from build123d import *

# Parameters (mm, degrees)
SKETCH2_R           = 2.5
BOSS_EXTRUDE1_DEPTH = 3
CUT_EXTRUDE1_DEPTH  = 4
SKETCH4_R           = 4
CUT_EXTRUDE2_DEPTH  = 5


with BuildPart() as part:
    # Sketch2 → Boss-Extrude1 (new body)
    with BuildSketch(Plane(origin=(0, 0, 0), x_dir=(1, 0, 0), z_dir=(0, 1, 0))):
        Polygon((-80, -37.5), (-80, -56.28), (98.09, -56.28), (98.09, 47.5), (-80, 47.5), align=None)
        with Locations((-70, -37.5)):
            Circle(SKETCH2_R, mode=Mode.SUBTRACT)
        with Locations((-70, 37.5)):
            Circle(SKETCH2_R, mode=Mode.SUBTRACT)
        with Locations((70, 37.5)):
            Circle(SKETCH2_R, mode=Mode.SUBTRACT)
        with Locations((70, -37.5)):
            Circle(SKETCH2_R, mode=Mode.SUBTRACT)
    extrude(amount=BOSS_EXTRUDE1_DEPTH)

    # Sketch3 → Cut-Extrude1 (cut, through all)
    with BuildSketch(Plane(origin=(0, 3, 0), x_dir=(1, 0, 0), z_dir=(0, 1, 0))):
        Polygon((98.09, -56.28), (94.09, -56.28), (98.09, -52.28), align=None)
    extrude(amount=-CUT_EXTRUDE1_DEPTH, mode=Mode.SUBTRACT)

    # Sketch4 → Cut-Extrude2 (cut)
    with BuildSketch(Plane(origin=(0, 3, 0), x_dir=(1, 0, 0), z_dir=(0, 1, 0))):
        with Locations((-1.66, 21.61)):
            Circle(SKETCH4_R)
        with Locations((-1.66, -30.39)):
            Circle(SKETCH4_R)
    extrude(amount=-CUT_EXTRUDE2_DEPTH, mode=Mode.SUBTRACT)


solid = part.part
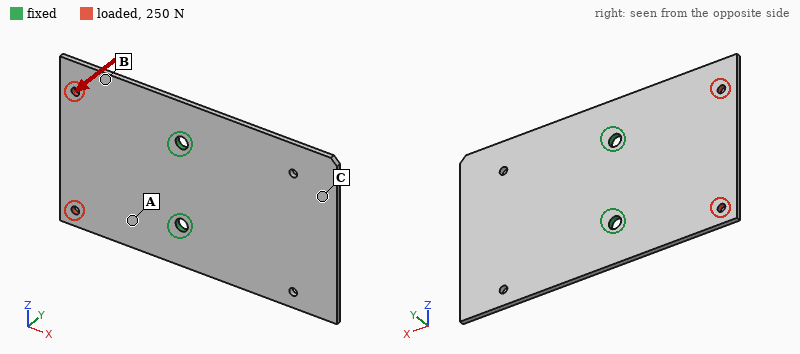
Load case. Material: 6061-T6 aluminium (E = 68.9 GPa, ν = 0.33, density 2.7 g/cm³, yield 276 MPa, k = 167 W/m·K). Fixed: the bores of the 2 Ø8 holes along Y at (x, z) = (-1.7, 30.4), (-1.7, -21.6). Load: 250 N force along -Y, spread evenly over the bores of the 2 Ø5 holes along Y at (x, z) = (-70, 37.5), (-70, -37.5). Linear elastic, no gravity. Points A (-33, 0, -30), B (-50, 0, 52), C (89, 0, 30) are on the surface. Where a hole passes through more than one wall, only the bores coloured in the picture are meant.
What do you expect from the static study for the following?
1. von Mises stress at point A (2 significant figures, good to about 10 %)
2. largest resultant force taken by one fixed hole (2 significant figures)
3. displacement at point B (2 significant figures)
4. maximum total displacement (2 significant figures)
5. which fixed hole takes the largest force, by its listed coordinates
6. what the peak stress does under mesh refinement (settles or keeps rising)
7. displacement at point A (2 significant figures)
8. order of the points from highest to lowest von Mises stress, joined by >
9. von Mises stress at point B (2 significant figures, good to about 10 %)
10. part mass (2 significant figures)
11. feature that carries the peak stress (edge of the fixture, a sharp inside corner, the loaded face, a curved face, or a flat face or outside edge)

55 MPa
140 N
0.85 mm
2.0 mm
(-1.7, -21.6)
keeps rising
0.44 mm
A > B > C
32 MPa
150 g
edge of the fixture
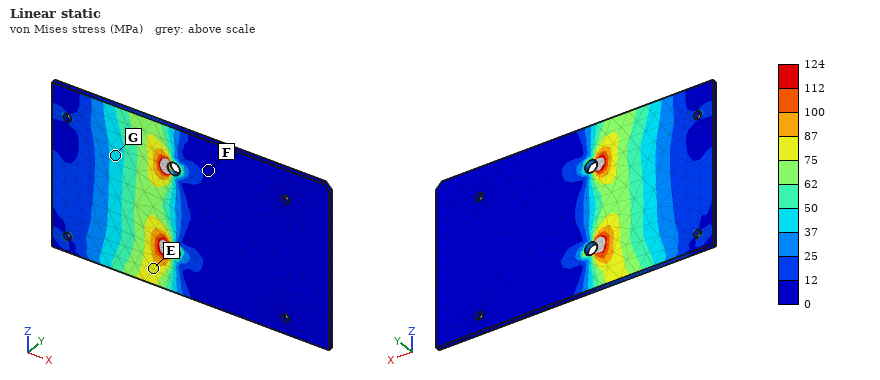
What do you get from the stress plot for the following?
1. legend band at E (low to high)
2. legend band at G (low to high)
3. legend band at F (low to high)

75 to 87 MPa
37 to 50 MPa
0 to 12 MPa
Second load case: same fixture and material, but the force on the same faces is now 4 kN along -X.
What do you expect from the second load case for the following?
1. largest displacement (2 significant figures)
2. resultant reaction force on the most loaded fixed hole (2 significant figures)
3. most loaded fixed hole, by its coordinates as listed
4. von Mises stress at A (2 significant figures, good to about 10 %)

31 µm
2.3 kN
(-1.7, -21.6)
19 MPa
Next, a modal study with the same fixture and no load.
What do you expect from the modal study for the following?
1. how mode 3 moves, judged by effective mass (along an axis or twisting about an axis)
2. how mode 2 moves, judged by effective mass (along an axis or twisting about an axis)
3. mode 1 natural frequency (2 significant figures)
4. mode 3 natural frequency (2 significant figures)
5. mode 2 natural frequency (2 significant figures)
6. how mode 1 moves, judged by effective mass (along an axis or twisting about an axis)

twisting about X
along Y
250 Hz
580 Hz
410 Hz
along Y
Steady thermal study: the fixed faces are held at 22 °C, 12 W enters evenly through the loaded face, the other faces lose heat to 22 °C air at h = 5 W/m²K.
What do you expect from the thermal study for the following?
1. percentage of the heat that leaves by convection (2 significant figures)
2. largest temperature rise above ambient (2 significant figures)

8.0 %
22 K
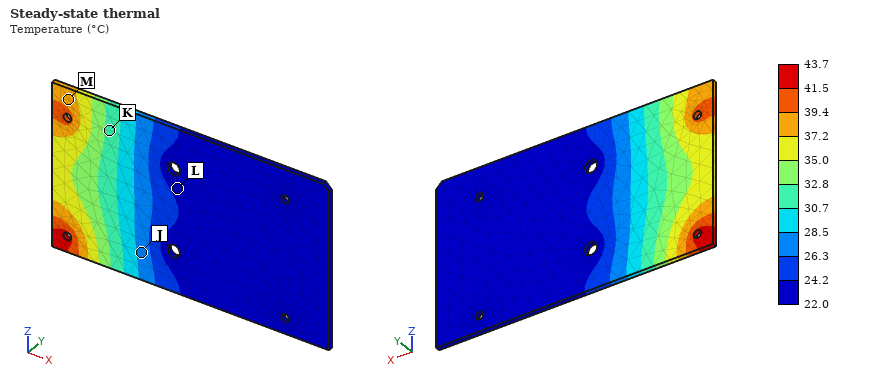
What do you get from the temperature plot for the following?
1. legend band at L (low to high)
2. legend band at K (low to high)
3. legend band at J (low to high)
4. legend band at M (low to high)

22.0 to 24.2 °C
30.7 to 32.8 °C
26.3 to 28.5 °C
37.2 to 39.4 °C
